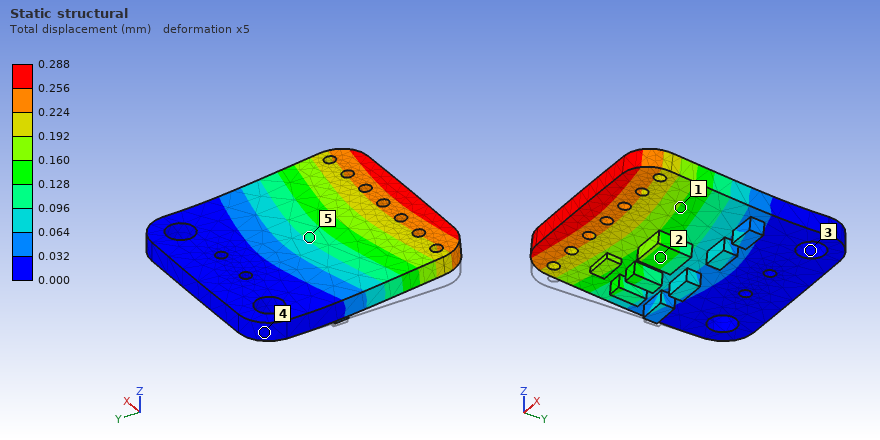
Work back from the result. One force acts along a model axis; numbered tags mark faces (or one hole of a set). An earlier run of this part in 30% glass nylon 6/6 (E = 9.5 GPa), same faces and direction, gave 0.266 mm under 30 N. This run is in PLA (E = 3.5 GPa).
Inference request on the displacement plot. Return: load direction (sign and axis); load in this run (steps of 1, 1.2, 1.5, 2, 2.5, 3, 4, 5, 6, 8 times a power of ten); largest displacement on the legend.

+Z
12 N
0.288 mm
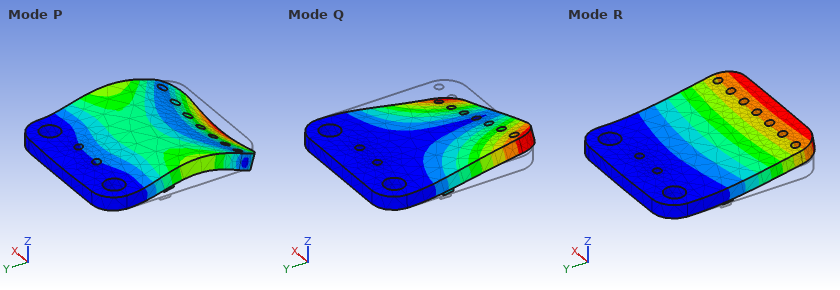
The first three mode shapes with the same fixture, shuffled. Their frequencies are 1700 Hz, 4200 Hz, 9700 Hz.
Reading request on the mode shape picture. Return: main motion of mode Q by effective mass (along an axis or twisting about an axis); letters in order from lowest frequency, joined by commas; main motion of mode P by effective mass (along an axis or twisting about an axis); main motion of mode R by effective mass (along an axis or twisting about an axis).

twisting about Y
R, Q, P
along Z
along Z
